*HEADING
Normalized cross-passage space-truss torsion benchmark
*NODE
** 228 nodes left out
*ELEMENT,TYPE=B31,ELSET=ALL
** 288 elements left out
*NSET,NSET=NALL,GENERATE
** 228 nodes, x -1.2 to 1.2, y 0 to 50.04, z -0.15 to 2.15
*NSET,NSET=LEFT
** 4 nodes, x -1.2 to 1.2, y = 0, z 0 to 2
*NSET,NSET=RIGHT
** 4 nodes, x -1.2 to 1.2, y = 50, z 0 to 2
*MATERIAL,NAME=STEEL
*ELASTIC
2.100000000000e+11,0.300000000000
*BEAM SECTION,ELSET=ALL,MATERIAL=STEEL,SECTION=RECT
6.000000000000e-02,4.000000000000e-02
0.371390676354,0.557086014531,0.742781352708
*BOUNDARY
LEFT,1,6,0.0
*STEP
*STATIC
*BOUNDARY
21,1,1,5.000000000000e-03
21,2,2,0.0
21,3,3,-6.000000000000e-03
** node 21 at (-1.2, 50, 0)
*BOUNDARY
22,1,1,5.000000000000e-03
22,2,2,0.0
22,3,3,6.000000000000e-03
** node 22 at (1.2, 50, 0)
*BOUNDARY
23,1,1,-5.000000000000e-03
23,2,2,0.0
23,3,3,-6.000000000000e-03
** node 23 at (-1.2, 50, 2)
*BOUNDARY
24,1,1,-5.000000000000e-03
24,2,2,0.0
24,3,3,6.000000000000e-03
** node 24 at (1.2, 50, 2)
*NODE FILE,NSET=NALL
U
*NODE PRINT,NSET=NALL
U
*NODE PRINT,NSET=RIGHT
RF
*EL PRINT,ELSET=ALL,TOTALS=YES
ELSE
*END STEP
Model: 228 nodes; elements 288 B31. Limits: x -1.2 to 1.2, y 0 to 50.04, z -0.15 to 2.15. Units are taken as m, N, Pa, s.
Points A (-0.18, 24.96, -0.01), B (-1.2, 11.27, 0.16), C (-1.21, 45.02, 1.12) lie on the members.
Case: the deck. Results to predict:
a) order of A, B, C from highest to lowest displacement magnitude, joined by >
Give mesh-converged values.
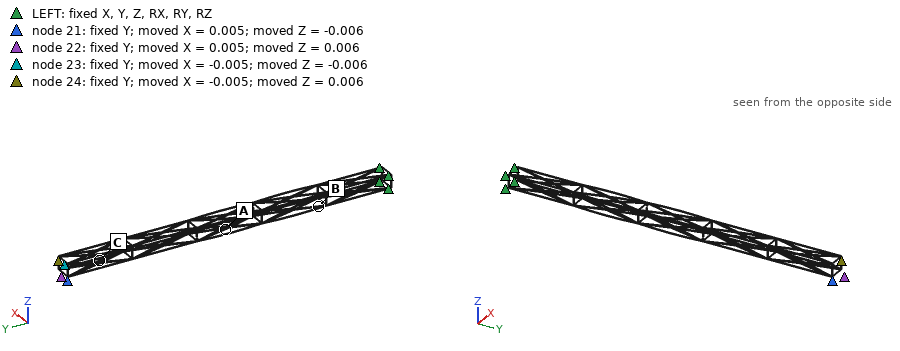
C > B > A
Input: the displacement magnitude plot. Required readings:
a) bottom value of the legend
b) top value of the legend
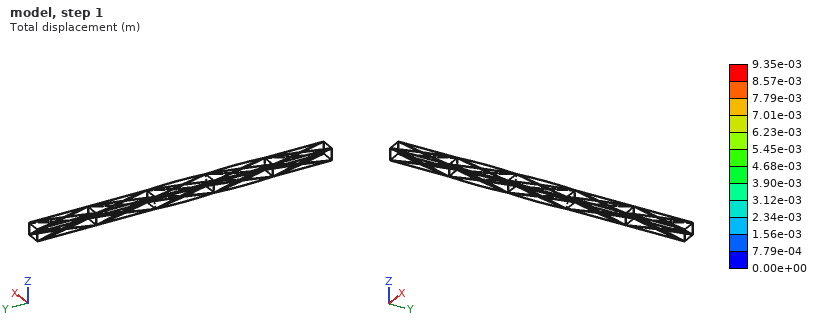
0.00e+00 m
9.35e-03 m
